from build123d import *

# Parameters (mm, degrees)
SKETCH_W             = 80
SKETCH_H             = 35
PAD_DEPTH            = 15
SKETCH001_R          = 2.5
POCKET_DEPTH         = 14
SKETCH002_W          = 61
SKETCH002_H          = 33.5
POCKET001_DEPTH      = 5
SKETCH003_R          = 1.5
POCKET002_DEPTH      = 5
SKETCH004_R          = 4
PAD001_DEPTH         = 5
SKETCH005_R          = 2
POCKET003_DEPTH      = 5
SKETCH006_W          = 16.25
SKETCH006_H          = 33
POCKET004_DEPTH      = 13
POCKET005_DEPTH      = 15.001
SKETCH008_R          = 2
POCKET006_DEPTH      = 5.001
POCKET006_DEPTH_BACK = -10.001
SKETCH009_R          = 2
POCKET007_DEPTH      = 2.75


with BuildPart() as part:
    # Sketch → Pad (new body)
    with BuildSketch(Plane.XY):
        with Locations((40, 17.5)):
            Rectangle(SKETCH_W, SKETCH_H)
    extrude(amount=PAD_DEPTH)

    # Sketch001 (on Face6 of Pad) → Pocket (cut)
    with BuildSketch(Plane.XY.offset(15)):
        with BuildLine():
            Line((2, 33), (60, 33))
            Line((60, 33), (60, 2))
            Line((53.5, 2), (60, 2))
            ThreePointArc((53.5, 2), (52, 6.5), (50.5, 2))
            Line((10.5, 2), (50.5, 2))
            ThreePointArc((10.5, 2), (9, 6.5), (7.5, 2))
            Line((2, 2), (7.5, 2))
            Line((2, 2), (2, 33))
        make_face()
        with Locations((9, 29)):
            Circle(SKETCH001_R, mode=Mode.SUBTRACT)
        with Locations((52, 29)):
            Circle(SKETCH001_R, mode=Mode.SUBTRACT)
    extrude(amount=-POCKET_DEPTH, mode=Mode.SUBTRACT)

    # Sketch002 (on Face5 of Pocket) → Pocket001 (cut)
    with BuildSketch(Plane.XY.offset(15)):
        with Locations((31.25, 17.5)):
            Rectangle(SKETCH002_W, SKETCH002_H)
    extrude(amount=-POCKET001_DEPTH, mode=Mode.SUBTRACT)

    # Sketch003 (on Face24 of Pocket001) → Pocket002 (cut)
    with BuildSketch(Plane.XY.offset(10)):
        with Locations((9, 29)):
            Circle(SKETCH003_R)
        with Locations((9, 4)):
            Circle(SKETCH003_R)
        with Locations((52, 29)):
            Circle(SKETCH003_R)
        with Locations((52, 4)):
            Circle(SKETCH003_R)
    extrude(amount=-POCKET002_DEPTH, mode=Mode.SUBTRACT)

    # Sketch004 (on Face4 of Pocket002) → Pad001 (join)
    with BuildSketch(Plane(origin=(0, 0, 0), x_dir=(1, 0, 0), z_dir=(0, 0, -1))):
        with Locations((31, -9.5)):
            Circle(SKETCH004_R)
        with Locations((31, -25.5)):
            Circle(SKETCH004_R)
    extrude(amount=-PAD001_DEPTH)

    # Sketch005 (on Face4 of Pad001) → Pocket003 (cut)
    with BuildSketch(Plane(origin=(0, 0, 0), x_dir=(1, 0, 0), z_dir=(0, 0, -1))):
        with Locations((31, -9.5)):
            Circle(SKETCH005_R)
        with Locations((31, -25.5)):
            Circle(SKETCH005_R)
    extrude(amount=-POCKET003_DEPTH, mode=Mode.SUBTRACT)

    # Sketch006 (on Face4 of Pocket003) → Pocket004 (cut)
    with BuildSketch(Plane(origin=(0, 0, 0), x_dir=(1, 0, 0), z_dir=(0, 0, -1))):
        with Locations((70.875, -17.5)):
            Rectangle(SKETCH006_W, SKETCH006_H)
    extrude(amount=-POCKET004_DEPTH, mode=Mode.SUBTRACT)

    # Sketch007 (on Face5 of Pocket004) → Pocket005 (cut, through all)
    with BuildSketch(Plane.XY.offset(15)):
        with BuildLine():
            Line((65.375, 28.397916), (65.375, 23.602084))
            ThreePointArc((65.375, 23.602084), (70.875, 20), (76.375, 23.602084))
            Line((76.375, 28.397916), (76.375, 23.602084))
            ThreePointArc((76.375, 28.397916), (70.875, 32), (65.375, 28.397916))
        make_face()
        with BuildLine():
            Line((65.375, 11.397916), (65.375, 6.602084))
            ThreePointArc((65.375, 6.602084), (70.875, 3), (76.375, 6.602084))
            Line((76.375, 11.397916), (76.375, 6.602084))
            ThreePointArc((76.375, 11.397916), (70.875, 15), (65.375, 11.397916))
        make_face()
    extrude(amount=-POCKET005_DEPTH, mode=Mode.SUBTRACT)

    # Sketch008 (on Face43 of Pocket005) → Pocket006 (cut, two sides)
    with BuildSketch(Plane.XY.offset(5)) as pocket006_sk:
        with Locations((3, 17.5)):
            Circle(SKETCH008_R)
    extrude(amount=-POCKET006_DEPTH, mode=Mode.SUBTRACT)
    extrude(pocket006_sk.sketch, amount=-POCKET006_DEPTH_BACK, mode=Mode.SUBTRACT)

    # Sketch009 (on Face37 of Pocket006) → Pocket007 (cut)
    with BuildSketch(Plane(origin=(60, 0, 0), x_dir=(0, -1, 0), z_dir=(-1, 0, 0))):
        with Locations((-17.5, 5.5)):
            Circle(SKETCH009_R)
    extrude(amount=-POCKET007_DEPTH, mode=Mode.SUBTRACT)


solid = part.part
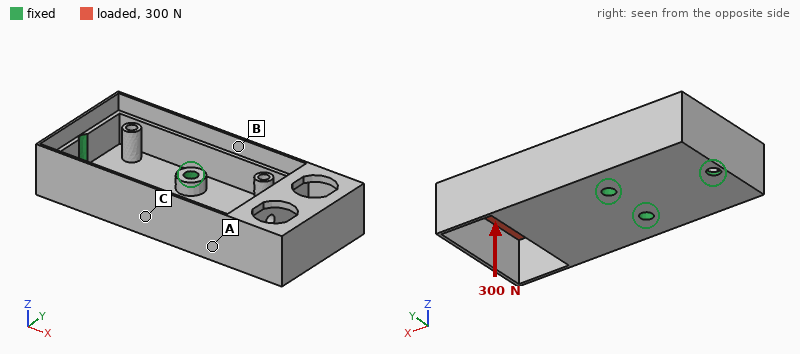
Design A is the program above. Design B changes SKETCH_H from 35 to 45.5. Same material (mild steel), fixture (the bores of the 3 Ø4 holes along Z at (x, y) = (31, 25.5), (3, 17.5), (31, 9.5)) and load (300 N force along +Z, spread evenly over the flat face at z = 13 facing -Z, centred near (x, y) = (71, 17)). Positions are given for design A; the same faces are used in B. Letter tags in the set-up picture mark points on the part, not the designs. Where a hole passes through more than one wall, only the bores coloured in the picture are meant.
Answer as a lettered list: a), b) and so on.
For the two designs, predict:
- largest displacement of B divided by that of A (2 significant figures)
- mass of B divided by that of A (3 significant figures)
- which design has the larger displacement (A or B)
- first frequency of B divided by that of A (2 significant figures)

a) 0.49
b) 2.41
c) A
d) 0.89
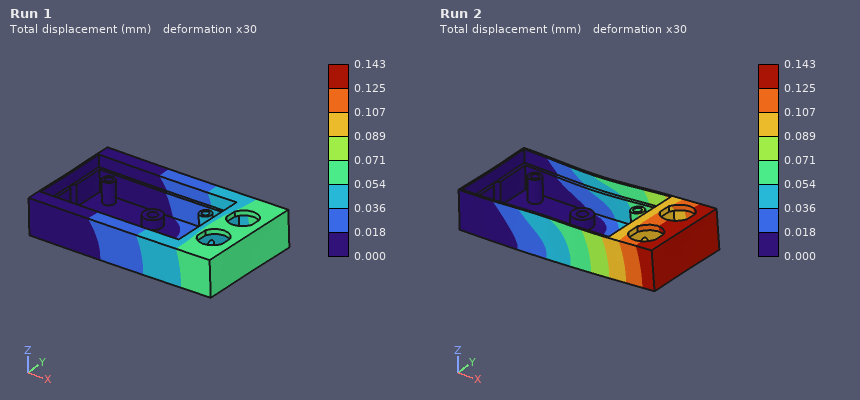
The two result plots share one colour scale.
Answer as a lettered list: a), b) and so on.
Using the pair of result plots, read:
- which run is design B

a) Run 1
